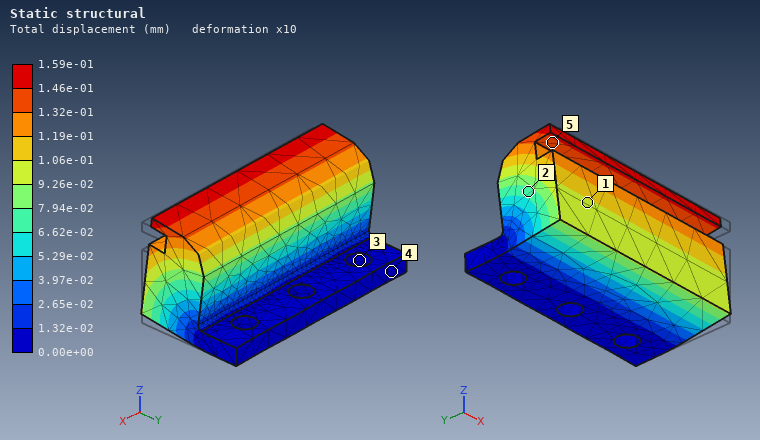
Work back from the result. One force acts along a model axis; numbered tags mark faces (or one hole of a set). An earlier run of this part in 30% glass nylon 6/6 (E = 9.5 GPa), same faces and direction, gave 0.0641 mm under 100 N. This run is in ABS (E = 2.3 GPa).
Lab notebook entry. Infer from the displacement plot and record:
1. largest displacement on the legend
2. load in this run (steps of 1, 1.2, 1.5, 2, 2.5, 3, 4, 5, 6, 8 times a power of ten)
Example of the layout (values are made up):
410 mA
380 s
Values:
1.59e-01 mm
60 N
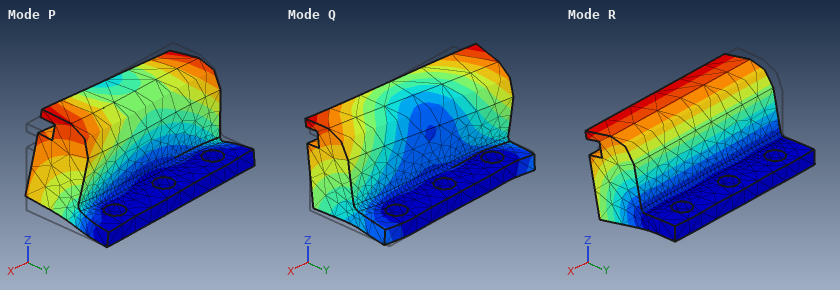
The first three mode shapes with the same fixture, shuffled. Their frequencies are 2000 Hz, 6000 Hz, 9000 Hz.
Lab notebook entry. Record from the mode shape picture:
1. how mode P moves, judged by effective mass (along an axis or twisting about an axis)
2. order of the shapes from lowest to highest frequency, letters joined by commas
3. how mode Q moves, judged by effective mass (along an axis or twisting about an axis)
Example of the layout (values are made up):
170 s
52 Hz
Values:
along X
R, P, Q
along X
